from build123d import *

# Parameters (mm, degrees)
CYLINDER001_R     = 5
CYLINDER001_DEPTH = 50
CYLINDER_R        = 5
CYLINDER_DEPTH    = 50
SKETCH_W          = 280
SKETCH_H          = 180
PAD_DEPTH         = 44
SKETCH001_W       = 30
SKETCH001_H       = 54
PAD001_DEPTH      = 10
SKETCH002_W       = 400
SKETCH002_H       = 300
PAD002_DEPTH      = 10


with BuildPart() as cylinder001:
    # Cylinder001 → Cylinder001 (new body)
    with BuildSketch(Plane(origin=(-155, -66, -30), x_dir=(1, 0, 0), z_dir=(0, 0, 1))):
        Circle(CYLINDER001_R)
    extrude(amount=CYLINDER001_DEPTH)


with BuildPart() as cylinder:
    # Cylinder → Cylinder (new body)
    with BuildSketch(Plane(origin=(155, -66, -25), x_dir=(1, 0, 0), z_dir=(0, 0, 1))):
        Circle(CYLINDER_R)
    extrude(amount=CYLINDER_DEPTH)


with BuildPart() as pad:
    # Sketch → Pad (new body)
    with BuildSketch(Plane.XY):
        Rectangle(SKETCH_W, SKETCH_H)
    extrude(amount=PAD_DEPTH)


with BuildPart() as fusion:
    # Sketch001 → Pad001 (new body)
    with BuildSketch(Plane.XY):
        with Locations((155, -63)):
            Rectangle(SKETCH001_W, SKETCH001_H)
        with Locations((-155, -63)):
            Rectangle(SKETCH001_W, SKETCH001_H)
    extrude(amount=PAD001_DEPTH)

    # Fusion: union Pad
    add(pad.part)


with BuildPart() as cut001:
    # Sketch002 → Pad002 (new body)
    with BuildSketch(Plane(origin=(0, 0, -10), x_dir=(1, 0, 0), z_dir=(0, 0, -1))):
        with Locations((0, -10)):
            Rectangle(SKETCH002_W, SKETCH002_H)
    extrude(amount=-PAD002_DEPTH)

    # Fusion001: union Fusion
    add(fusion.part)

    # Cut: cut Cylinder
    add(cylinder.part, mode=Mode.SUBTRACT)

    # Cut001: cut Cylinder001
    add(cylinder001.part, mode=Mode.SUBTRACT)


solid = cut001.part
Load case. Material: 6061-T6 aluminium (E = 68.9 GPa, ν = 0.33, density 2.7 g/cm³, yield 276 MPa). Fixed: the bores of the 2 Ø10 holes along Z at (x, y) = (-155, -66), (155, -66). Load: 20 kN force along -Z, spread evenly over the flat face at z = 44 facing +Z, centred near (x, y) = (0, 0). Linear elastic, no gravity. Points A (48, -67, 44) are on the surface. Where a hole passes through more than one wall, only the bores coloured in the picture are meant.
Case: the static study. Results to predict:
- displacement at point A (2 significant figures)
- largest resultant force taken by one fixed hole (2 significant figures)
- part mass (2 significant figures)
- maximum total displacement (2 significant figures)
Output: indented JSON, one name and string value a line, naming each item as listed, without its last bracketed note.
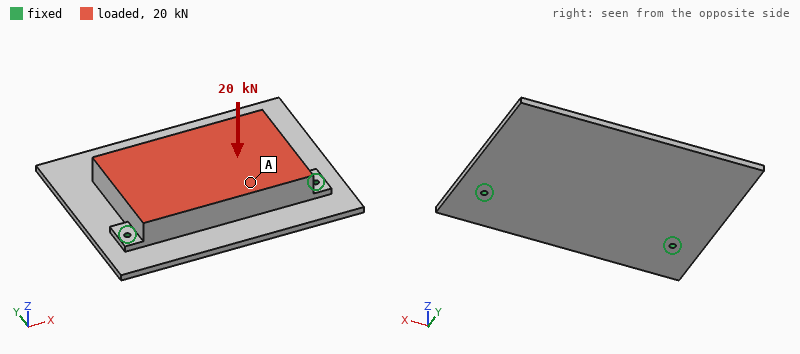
{
  "displacement at point A": "0.21 mm",
  "largest resultant force taken by one fixed hole": "12 kN",
  "part mass": "9.3 kg",
  "maximum total displacement": "1.1 mm"
}
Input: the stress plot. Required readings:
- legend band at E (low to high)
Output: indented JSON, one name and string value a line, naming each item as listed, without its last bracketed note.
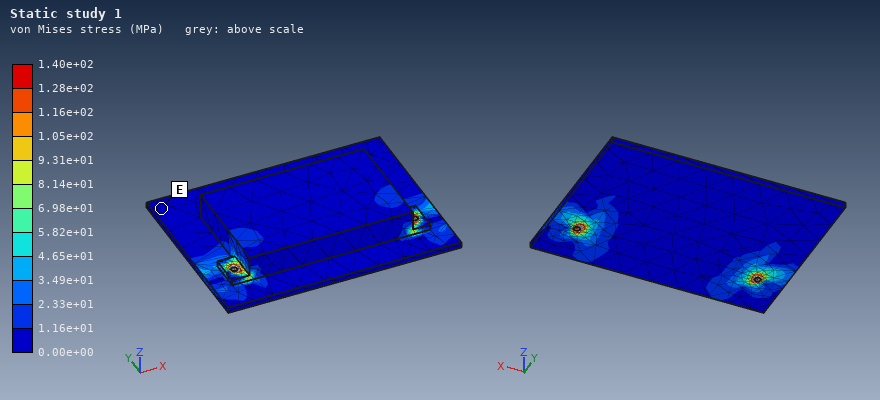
{
  "legend band at E": "0.00e+00 to 1.16e+01 MPa"
}
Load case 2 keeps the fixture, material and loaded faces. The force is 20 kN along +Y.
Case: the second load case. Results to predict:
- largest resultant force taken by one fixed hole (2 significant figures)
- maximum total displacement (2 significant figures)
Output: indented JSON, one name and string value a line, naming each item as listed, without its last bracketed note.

{
  "largest resultant force taken by one fixed hole": "10 kN",
  "maximum total displacement": "0.75 mm"
}
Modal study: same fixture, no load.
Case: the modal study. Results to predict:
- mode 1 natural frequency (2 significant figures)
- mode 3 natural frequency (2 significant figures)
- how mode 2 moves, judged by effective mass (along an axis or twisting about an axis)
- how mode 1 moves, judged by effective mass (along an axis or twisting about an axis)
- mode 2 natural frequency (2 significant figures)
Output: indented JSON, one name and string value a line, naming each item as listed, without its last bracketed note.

{
  "mode 1 natural frequency": "280 Hz",
  "mode 3 natural frequency": "1300 Hz",
  "how mode 2 moves, judged by effective mass": "twisting about Y",
  "how mode 1 moves, judged by effective mass": "along Z",
  "mode 2 natural frequency": "1000 Hz"
}
